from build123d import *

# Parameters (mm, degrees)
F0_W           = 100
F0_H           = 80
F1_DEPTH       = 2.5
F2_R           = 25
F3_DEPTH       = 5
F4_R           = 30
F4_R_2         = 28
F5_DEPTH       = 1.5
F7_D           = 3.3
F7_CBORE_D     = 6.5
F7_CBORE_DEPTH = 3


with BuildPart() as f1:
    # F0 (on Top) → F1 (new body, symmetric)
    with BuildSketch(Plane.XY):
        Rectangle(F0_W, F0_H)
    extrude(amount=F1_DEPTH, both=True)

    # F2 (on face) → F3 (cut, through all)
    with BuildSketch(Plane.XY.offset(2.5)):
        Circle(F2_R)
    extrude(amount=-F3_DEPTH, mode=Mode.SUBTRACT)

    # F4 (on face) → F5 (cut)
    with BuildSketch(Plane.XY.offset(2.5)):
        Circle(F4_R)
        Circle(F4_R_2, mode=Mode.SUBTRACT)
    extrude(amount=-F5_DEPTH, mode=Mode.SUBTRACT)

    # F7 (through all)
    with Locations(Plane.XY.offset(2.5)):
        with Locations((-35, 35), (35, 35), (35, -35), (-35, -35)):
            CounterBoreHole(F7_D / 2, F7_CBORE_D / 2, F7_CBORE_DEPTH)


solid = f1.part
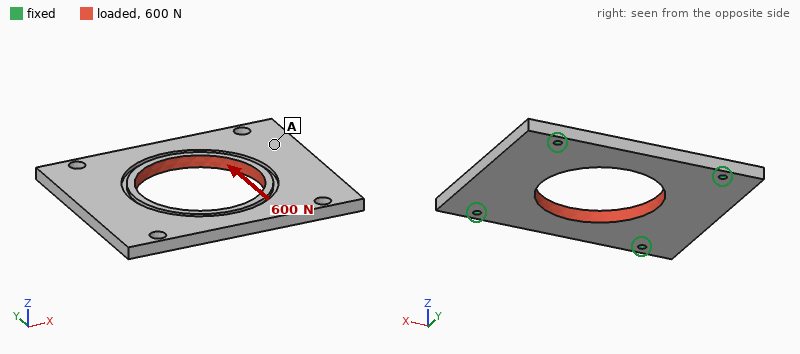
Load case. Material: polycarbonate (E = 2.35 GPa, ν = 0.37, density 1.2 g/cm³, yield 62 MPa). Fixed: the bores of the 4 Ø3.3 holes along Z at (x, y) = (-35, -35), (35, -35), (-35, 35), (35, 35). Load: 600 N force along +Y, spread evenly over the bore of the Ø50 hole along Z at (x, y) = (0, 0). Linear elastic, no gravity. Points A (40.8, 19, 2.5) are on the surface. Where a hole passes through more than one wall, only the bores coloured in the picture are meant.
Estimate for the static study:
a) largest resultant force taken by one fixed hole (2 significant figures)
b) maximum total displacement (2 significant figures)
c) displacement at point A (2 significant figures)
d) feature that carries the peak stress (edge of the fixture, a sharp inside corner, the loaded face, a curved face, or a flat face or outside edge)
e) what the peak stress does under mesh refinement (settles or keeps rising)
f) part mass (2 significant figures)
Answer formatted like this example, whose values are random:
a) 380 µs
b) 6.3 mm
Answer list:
a) 160 N
b) 77 µm
c) 24 µm
d) edge of the fixture
e) keeps rising
f) 35 g
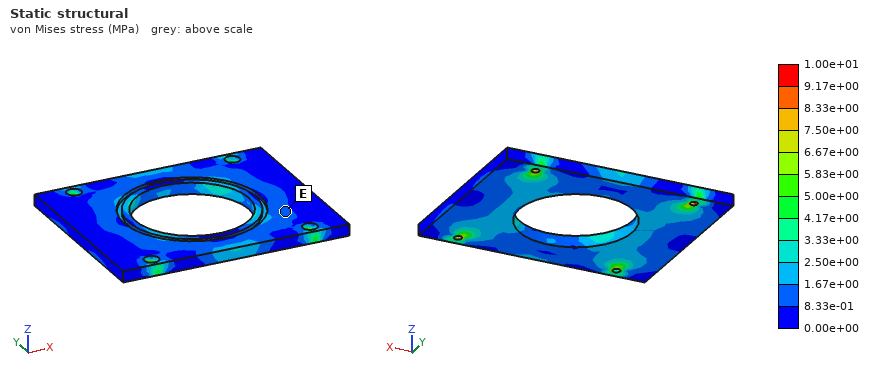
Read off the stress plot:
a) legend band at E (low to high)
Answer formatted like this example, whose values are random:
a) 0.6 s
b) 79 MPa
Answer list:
a) 8.33e-01 to 1.67e+00 MPa
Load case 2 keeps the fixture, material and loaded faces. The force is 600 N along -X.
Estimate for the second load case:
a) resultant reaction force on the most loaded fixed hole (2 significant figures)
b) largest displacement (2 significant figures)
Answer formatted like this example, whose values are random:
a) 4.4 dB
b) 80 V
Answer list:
a) 150 N
b) 67 µm
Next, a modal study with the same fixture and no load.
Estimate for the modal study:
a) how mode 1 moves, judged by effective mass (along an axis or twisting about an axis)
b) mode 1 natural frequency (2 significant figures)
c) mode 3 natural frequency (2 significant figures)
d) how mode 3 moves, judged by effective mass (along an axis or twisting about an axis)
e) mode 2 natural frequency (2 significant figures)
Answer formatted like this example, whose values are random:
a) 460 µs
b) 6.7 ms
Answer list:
a) along Z
b) 910 Hz
c) 1000 Hz
d) twisting about Y
e) 950 Hz
